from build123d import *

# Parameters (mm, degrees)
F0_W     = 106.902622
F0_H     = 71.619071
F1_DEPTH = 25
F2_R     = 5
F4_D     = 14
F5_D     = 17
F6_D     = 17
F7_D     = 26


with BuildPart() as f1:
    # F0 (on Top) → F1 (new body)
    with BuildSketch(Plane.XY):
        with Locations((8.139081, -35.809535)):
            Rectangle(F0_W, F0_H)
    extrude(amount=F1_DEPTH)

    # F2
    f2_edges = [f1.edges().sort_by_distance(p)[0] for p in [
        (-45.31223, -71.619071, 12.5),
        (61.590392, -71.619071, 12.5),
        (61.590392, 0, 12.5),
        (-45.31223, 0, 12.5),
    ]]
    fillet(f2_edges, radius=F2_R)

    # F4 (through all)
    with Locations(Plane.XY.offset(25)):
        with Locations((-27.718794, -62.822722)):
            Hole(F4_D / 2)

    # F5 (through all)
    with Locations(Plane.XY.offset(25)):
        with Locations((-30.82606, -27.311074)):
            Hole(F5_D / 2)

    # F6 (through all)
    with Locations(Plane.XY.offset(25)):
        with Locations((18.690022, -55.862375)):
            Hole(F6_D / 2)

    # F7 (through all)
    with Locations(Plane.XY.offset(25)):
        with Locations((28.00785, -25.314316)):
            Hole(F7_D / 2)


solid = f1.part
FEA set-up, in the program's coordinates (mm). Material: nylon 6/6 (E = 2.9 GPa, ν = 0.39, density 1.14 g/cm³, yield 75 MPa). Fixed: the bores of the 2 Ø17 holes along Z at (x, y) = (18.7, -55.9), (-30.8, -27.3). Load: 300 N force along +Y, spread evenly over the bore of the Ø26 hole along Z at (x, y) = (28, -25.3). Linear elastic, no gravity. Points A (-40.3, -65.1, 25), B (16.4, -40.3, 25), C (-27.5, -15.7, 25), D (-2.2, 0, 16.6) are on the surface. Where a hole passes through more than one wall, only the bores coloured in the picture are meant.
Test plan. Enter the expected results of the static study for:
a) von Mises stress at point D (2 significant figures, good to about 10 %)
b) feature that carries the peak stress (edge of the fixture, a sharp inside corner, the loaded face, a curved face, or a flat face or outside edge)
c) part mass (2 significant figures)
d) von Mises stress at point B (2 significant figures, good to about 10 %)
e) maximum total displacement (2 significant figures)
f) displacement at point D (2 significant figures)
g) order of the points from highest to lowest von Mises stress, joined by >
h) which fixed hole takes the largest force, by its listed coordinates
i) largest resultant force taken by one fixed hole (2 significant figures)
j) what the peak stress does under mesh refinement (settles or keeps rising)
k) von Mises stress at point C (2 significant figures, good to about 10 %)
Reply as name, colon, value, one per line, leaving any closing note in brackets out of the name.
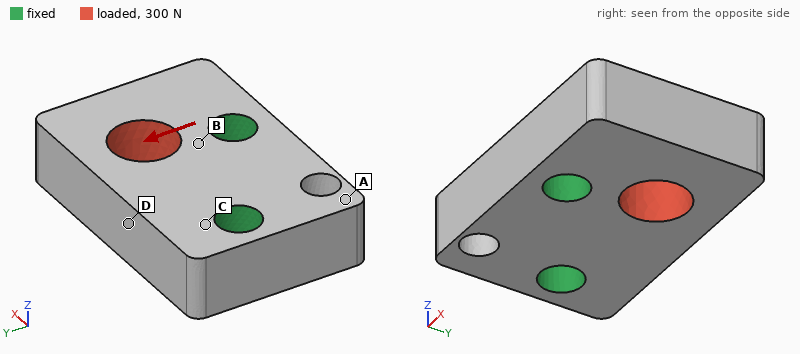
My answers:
von Mises stress at point D: 0.23 MPa
feature that carries the peak stress: edge of the fixture
part mass: 190 g
von Mises stress at point B: 0.47 MPa
maximum total displacement: 9.8 µm
displacement at point D: 3.1 µm
order of the points from highest to lowest von Mises stress, joined by >: B > D > C > A
which fixed hole takes the largest force, by its listed coordinates: (18.7, -55.9)
largest resultant force taken by one fixed hole: 290 N
what the peak stress does under mesh refinement: keeps rising
von Mises stress at point C: 0.13 MPa
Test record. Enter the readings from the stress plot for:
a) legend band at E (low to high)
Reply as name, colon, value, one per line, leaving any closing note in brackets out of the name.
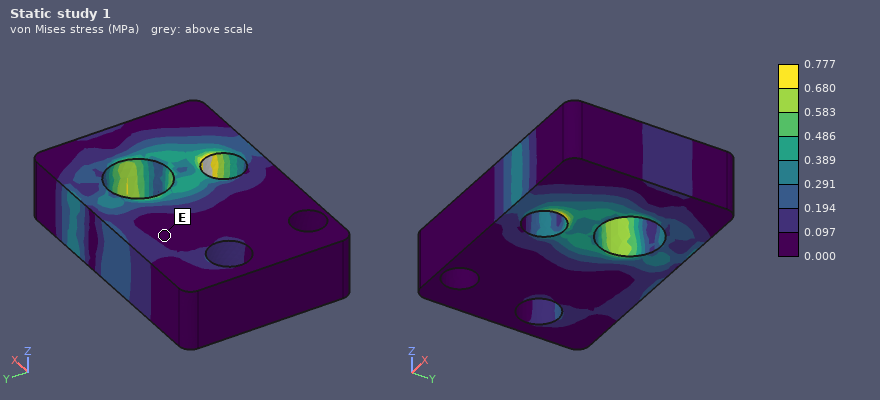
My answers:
legend band at E: 0.000 to 0.097 MPa
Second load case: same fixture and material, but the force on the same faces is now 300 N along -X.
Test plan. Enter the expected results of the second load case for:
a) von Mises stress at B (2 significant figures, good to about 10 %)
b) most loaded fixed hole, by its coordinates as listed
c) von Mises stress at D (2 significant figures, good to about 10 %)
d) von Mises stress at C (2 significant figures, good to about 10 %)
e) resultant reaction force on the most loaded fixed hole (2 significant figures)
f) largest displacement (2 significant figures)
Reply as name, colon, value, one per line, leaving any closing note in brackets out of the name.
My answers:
von Mises stress at B: 0.30 MPa
most loaded fixed hole, by its coordinates as listed: (-30.8, -27.3)
von Mises stress at D: 0.25 MPa
von Mises stress at C: 0.23 MPa
resultant reaction force on the most loaded fixed hole: 170 N
largest displacement: 7.5 µm
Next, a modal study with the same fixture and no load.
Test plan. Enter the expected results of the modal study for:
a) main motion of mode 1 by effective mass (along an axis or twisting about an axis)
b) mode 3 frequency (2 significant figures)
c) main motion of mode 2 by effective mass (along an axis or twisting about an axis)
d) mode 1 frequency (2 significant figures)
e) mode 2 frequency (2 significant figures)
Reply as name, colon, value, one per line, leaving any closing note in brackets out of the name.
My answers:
main motion of mode 1 by effective mass: along Z
mode 3 frequency: 3300 Hz
main motion of mode 2 by effective mass: along Y
mode 1 frequency: 1700 Hz
mode 2 frequency: 2900 Hz
